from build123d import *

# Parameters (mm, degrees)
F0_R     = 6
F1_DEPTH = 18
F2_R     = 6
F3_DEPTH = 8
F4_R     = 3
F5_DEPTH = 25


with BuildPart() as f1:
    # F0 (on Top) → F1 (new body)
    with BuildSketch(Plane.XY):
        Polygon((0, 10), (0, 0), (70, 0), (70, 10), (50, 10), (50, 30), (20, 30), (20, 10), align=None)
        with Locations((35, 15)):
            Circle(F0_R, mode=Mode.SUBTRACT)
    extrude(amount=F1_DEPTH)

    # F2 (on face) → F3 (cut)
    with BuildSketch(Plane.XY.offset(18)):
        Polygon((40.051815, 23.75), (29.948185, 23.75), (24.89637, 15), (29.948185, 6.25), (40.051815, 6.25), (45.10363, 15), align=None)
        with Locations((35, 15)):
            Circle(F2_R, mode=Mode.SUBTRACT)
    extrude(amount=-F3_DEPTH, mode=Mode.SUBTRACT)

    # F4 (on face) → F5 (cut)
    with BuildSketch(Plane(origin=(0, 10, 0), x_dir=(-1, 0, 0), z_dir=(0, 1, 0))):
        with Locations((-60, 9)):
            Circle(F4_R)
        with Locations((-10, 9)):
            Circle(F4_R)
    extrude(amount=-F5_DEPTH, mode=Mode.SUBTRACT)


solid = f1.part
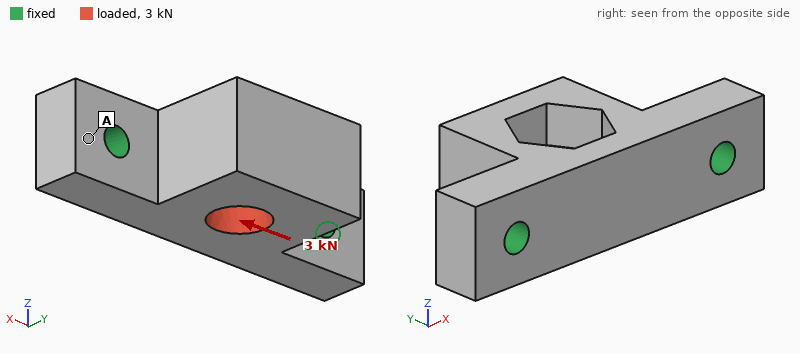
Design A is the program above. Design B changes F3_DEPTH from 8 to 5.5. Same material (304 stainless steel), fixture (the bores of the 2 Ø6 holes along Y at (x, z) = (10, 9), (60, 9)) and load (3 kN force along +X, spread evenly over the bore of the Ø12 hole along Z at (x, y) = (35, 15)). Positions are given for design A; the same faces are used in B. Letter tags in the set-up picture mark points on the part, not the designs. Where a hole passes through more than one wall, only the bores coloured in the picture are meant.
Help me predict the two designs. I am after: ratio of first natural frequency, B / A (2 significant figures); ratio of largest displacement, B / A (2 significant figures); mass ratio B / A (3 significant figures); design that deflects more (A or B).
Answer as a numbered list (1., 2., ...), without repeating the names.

1. 0.99
2. 0.92
3. 1.02
4. A
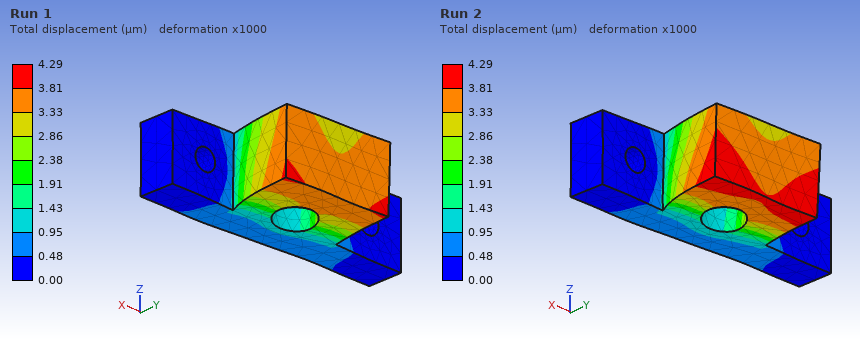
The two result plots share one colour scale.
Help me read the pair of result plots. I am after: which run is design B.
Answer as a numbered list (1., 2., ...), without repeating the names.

1. Run 1
